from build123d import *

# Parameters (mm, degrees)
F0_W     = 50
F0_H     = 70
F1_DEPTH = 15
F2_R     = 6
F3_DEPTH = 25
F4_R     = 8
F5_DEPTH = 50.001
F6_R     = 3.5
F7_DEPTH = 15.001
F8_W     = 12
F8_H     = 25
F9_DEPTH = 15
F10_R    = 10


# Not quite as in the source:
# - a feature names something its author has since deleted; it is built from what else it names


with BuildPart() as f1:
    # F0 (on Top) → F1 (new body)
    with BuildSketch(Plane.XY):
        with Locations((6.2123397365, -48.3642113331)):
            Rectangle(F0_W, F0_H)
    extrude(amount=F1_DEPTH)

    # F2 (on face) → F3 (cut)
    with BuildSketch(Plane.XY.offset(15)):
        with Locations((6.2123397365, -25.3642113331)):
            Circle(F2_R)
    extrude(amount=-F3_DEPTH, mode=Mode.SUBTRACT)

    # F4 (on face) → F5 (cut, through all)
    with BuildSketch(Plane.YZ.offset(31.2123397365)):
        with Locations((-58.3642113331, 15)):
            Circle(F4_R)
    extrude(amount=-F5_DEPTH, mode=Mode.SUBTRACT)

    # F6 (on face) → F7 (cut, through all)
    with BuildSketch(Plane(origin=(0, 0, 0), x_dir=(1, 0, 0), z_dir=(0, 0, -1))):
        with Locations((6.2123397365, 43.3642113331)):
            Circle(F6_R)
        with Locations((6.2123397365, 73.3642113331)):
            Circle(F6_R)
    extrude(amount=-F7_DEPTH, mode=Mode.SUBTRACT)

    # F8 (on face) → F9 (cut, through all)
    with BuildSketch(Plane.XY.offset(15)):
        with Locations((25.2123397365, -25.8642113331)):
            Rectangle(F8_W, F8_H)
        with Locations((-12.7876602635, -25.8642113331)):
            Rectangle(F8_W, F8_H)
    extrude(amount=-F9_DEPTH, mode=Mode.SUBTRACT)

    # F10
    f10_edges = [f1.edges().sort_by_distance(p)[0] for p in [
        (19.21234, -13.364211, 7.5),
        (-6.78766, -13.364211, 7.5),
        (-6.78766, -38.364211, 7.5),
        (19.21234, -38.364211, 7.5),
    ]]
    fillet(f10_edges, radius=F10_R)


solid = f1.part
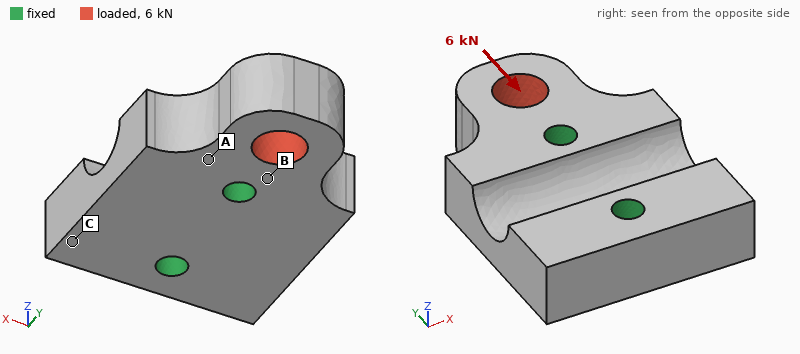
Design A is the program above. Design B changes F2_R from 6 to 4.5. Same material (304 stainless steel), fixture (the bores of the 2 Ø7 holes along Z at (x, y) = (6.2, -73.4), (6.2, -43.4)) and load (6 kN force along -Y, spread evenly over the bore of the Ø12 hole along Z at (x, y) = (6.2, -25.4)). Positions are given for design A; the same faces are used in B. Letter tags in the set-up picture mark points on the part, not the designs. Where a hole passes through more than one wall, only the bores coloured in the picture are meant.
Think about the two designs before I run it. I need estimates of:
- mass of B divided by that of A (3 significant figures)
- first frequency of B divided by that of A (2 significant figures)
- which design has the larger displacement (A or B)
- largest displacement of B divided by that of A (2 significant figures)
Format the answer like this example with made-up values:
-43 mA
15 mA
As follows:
1.02
1.0
A
0.79
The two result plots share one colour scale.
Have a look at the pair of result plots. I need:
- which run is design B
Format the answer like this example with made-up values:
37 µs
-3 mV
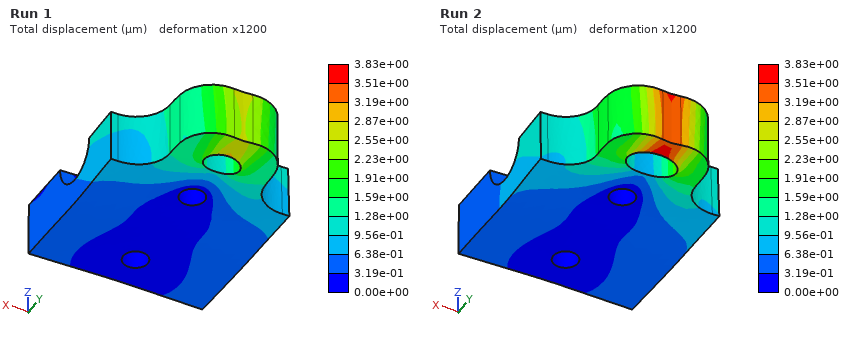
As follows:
Run 1
